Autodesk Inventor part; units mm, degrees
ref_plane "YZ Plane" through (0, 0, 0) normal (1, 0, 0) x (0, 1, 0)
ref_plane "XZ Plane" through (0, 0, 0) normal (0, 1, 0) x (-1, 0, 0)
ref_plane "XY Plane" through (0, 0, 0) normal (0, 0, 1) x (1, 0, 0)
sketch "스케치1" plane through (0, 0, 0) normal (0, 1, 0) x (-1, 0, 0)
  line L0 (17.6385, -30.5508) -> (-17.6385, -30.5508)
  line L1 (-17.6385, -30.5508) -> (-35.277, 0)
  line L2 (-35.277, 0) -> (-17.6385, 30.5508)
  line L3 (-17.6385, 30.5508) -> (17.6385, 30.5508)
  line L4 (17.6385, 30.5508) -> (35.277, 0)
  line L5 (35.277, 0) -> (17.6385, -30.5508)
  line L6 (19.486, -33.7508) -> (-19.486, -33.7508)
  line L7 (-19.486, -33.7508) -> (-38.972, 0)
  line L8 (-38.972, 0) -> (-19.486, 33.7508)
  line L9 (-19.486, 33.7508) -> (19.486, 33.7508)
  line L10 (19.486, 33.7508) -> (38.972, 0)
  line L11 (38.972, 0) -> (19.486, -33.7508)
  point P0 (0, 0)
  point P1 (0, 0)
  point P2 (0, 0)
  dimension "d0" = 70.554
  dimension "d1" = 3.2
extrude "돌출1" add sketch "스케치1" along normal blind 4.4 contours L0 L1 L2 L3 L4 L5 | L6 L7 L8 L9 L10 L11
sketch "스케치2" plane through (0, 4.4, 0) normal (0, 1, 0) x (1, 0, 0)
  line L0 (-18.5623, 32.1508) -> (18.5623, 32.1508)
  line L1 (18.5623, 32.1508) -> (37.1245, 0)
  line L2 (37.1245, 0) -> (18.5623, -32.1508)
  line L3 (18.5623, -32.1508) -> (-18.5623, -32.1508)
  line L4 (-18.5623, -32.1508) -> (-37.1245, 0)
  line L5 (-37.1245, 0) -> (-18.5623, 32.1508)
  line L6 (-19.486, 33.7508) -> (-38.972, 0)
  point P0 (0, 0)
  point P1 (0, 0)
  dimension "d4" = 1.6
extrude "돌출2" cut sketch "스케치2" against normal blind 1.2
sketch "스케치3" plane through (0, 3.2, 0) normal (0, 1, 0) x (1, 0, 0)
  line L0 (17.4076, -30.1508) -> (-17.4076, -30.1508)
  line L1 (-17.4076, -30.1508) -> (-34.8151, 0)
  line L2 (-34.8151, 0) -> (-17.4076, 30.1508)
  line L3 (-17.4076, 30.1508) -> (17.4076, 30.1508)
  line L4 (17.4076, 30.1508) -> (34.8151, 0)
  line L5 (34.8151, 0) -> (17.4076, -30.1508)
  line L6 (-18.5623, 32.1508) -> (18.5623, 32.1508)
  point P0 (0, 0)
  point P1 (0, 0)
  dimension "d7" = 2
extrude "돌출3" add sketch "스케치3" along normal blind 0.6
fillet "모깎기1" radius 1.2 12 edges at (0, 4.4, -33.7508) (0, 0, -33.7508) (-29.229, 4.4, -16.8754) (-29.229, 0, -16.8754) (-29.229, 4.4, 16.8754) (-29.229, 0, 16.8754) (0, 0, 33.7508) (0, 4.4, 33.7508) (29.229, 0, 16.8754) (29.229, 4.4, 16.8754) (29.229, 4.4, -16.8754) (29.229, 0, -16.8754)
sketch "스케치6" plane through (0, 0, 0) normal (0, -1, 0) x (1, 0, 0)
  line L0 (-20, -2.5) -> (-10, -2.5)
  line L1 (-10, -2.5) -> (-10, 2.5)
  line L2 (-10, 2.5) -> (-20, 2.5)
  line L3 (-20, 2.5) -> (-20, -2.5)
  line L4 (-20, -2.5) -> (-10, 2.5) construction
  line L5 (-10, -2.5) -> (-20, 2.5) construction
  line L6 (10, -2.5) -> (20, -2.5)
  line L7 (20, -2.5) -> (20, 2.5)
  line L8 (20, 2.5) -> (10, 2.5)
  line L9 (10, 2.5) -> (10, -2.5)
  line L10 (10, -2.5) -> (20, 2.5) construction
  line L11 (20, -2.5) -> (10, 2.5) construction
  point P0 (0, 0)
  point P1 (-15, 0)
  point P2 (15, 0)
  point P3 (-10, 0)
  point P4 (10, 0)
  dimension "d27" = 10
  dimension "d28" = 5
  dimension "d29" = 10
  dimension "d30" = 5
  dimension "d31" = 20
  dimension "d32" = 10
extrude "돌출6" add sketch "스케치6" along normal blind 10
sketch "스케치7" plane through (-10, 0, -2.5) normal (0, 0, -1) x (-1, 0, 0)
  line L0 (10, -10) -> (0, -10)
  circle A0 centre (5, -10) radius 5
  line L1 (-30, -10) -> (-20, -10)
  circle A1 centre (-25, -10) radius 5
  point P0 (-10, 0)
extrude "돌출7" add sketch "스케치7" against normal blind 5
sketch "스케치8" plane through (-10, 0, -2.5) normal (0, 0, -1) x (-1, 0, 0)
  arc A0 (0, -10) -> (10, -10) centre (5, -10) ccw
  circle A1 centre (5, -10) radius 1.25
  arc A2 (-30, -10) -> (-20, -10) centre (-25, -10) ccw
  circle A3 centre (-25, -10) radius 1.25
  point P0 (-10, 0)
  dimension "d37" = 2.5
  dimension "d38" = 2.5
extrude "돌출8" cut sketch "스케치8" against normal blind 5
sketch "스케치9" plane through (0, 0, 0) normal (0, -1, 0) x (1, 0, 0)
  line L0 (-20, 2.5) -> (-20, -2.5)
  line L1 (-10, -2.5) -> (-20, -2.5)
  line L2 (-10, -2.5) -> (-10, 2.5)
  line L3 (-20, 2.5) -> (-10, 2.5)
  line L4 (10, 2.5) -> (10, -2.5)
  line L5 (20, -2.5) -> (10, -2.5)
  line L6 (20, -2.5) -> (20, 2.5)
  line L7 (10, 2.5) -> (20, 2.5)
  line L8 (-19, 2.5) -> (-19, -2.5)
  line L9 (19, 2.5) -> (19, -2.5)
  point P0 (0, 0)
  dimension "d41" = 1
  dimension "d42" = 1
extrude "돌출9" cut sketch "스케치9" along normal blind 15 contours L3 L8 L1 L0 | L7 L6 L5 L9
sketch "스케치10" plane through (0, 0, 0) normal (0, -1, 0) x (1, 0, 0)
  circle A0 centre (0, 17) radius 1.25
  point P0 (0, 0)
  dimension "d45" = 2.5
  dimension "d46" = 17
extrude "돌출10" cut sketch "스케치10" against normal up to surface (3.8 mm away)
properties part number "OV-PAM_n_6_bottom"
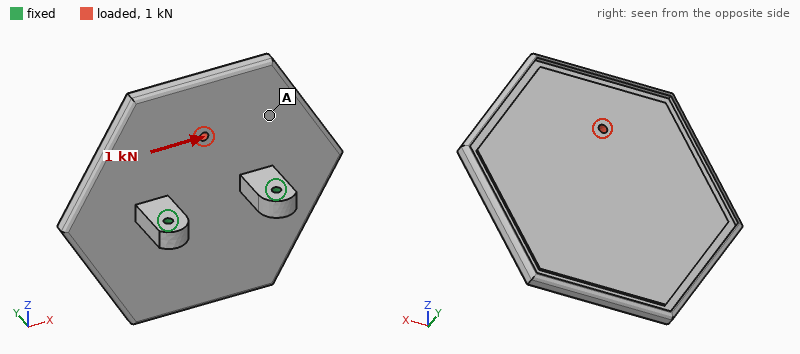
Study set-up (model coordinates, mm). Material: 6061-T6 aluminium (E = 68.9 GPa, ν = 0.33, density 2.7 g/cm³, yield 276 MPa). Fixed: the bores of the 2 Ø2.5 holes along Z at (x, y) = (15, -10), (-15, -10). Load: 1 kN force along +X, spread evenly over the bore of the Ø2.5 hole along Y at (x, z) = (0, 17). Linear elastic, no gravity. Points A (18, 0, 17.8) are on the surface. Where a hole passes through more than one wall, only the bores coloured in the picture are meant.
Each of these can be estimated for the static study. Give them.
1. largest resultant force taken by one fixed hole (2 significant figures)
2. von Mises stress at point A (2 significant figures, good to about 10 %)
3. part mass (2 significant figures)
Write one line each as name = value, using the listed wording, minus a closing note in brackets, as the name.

largest resultant force taken by one fixed hole = 740 N
von Mises stress at point A = 16 MPa
part mass = 43 g
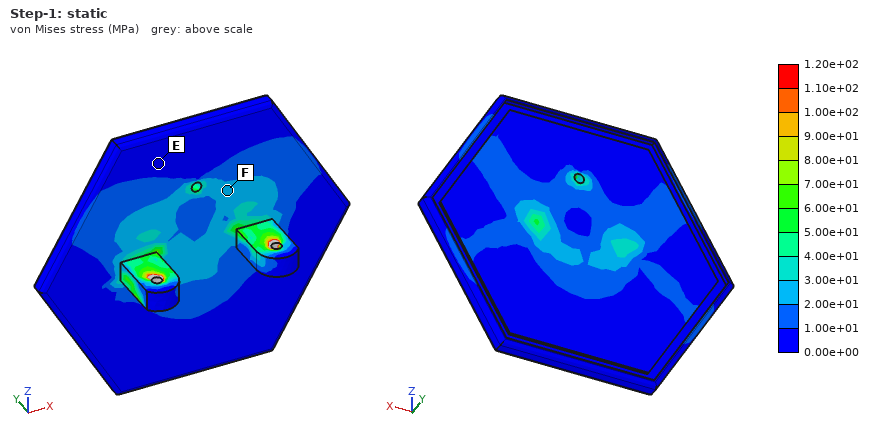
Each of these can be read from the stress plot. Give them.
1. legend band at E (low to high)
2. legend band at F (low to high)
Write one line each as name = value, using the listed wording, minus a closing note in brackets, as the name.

legend band at E = 0.00e+00 to 1.00e+01 MPa
legend band at F = 2.00e+01 to 3.00e+01 MPa
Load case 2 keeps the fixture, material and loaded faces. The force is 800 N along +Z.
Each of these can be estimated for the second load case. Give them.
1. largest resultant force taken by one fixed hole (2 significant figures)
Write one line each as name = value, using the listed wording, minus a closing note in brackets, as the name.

largest resultant force taken by one fixed hole = 400 N
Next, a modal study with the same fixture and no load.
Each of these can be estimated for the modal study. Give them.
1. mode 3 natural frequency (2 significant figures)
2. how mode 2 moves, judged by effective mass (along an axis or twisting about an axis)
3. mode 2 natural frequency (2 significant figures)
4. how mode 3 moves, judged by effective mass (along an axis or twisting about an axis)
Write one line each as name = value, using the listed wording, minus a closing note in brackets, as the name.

mode 3 natural frequency = 3300 Hz
how mode 2 moves, judged by effective mass = twisting about Y
mode 2 natural frequency = 3000 Hz
how mode 3 moves, judged by effective mass = along Y
